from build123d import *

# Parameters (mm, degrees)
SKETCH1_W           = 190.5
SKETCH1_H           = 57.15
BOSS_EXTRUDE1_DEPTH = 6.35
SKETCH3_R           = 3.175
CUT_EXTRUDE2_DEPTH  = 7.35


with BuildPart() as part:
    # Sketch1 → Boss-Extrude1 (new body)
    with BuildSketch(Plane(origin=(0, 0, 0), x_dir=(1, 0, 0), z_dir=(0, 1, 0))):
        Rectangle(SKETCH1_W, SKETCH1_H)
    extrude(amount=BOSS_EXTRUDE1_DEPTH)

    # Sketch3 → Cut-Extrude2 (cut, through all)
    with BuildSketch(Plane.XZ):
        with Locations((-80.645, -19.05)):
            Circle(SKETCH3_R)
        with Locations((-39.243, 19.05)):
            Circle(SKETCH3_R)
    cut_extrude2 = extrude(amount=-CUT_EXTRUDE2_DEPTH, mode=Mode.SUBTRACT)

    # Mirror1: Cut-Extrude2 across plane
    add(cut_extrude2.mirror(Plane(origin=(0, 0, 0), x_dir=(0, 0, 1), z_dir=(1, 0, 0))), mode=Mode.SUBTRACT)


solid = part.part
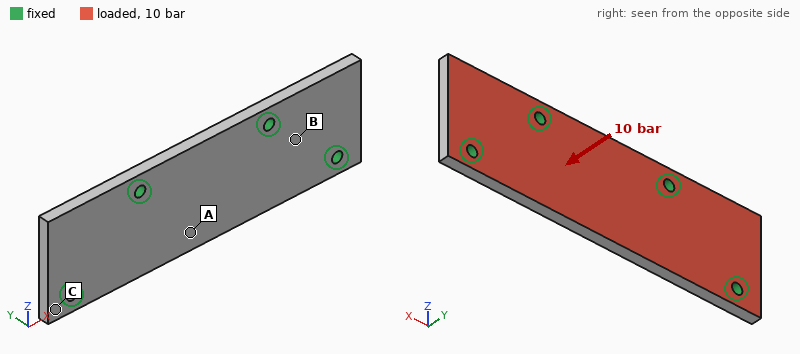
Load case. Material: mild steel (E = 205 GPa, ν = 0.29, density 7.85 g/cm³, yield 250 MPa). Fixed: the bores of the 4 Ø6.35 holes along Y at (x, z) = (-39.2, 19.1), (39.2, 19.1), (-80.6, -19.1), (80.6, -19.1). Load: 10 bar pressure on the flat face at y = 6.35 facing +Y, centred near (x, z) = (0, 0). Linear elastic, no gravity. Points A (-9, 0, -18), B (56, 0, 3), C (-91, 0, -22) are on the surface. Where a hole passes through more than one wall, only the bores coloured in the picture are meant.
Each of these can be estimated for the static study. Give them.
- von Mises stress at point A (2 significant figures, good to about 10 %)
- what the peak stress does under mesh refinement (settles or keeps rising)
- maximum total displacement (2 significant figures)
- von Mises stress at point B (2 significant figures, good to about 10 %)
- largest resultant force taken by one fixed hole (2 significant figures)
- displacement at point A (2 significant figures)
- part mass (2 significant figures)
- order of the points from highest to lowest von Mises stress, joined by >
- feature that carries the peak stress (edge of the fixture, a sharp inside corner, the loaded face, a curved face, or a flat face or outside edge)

51 MPa
keeps rising
0.15 mm
70 MPa
3.3 kN
0.12 mm
540 g
B > A > C
edge of the fixture
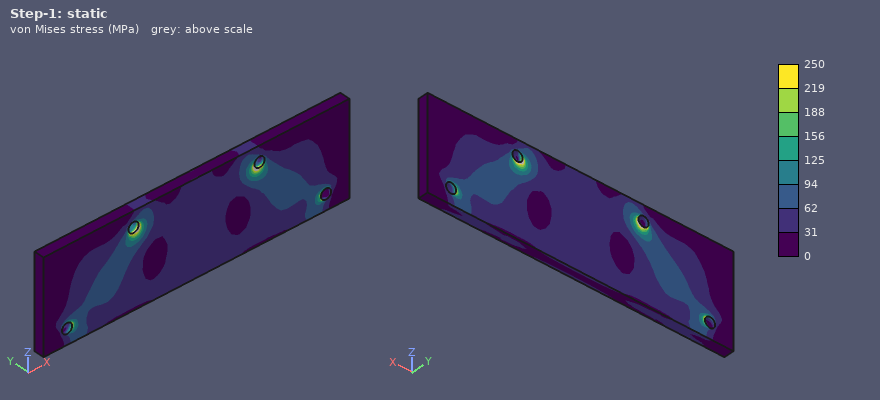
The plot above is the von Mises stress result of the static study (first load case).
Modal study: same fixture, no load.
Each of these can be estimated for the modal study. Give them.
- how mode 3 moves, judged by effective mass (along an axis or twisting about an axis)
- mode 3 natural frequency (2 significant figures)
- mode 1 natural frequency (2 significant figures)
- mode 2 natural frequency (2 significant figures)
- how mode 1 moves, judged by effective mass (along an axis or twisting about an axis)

along Y
3900 Hz
2400 Hz
3800 Hz
along Y
